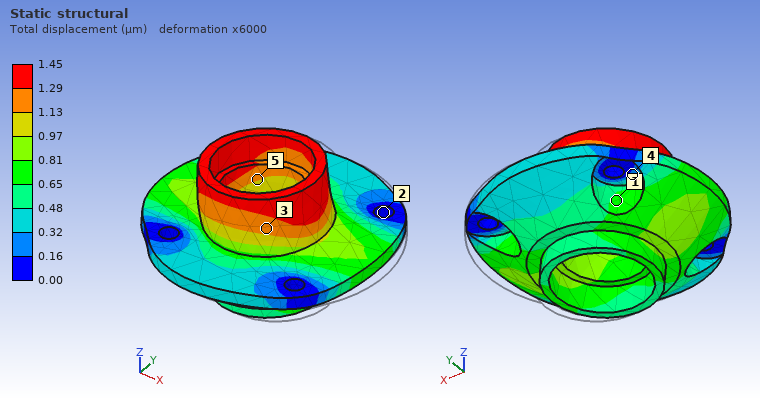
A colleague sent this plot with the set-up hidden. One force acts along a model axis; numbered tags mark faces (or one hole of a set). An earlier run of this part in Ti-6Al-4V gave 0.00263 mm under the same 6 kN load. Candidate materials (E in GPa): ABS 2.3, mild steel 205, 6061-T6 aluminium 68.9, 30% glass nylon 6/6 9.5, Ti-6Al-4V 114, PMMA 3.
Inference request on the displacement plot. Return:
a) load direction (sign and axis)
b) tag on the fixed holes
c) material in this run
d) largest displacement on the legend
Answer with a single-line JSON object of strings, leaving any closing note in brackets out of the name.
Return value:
{"load direction": "-X", "tag on the fixed holes": "2", "material in this run": "mild steel", "largest displacement on the legend": "1.45 µm"}
